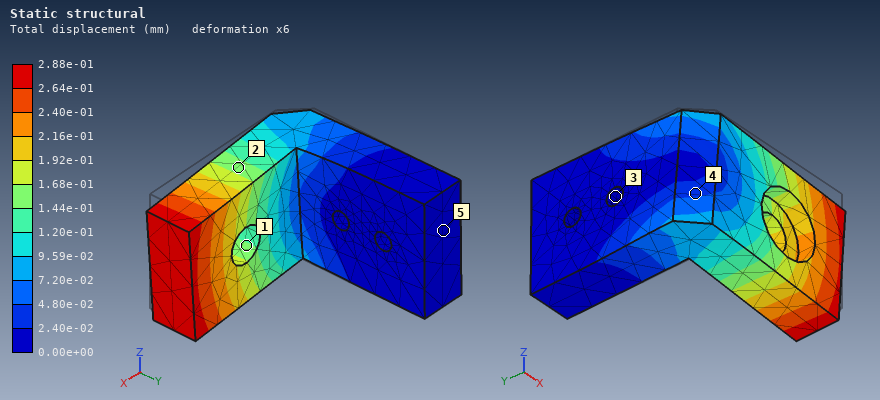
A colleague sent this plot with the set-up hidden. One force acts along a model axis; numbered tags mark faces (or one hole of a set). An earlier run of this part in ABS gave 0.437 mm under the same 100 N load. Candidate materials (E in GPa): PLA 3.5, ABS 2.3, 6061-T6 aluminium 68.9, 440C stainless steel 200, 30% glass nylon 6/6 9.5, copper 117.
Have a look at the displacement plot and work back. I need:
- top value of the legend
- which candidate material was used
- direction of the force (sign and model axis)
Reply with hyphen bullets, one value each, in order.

- 2.88e-01 mm
- PLA
- -Z
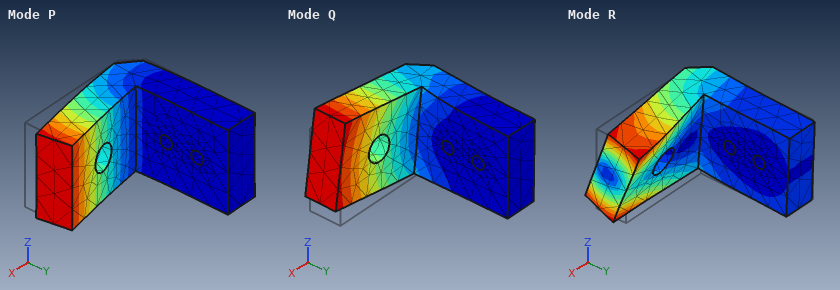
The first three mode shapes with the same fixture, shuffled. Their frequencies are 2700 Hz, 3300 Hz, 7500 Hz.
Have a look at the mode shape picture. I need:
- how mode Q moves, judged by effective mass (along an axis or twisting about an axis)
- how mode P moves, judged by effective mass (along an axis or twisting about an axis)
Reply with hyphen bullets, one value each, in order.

- along Z
- along Y
